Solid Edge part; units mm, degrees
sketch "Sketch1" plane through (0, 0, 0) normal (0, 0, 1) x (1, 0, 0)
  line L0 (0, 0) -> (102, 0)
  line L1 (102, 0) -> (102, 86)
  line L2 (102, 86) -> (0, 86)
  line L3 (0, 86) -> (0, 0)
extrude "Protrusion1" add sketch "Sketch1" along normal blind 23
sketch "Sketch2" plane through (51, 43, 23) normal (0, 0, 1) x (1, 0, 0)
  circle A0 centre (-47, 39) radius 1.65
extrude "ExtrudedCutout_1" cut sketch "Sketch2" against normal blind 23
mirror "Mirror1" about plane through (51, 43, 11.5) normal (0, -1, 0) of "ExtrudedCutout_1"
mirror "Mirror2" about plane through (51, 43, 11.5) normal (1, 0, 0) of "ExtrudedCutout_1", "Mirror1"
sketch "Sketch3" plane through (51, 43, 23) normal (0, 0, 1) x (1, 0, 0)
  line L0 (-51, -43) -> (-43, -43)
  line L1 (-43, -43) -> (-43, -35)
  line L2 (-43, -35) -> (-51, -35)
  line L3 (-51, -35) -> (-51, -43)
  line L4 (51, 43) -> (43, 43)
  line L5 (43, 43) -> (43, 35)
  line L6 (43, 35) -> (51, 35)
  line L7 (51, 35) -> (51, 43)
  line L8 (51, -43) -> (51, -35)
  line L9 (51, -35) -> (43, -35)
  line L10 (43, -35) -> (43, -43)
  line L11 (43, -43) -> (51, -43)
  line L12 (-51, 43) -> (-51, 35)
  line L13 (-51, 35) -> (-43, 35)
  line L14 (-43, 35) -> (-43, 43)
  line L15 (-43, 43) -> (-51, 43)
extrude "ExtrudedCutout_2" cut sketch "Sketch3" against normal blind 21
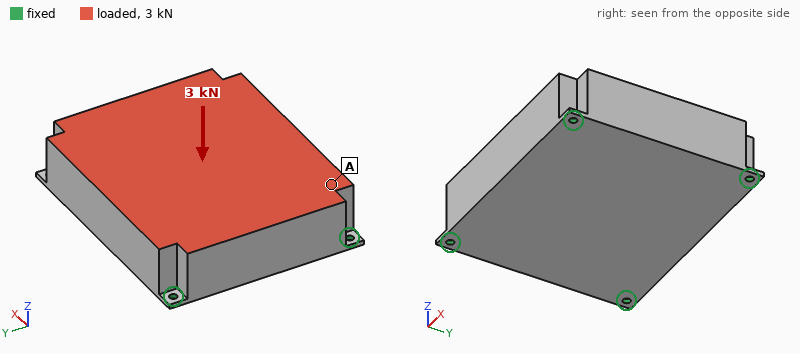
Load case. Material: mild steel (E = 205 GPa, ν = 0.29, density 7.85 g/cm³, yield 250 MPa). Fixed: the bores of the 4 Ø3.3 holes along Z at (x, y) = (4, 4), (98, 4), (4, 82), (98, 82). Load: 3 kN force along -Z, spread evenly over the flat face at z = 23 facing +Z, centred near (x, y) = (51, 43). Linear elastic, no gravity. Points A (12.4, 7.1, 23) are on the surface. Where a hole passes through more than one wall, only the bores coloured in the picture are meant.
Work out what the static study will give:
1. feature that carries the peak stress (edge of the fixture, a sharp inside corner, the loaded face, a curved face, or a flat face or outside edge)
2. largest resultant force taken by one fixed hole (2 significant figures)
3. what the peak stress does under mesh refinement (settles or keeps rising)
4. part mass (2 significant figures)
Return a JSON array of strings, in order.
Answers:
["edge of the fixture", "880 N", "keeps rising", "1.5 kg"]
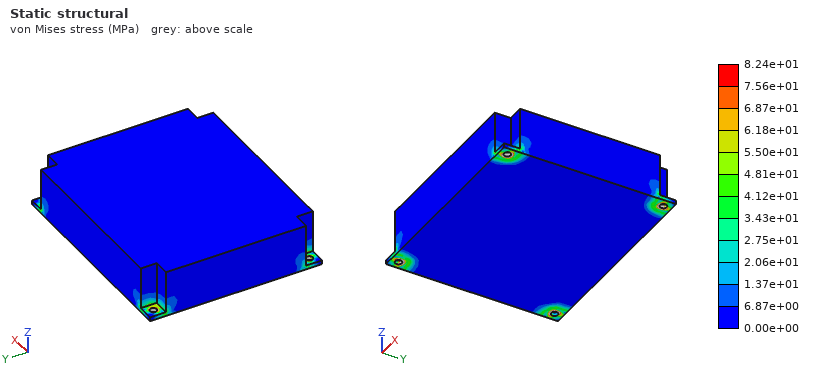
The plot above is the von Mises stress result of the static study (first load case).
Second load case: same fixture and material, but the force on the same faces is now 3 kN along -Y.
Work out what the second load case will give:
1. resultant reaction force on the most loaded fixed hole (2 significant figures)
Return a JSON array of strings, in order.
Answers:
["910 N"]
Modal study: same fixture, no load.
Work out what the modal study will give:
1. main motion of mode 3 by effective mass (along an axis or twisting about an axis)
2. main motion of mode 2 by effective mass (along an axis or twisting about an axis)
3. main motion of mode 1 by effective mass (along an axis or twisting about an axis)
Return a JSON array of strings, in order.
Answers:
["along X", "along Y", "along Z"]
